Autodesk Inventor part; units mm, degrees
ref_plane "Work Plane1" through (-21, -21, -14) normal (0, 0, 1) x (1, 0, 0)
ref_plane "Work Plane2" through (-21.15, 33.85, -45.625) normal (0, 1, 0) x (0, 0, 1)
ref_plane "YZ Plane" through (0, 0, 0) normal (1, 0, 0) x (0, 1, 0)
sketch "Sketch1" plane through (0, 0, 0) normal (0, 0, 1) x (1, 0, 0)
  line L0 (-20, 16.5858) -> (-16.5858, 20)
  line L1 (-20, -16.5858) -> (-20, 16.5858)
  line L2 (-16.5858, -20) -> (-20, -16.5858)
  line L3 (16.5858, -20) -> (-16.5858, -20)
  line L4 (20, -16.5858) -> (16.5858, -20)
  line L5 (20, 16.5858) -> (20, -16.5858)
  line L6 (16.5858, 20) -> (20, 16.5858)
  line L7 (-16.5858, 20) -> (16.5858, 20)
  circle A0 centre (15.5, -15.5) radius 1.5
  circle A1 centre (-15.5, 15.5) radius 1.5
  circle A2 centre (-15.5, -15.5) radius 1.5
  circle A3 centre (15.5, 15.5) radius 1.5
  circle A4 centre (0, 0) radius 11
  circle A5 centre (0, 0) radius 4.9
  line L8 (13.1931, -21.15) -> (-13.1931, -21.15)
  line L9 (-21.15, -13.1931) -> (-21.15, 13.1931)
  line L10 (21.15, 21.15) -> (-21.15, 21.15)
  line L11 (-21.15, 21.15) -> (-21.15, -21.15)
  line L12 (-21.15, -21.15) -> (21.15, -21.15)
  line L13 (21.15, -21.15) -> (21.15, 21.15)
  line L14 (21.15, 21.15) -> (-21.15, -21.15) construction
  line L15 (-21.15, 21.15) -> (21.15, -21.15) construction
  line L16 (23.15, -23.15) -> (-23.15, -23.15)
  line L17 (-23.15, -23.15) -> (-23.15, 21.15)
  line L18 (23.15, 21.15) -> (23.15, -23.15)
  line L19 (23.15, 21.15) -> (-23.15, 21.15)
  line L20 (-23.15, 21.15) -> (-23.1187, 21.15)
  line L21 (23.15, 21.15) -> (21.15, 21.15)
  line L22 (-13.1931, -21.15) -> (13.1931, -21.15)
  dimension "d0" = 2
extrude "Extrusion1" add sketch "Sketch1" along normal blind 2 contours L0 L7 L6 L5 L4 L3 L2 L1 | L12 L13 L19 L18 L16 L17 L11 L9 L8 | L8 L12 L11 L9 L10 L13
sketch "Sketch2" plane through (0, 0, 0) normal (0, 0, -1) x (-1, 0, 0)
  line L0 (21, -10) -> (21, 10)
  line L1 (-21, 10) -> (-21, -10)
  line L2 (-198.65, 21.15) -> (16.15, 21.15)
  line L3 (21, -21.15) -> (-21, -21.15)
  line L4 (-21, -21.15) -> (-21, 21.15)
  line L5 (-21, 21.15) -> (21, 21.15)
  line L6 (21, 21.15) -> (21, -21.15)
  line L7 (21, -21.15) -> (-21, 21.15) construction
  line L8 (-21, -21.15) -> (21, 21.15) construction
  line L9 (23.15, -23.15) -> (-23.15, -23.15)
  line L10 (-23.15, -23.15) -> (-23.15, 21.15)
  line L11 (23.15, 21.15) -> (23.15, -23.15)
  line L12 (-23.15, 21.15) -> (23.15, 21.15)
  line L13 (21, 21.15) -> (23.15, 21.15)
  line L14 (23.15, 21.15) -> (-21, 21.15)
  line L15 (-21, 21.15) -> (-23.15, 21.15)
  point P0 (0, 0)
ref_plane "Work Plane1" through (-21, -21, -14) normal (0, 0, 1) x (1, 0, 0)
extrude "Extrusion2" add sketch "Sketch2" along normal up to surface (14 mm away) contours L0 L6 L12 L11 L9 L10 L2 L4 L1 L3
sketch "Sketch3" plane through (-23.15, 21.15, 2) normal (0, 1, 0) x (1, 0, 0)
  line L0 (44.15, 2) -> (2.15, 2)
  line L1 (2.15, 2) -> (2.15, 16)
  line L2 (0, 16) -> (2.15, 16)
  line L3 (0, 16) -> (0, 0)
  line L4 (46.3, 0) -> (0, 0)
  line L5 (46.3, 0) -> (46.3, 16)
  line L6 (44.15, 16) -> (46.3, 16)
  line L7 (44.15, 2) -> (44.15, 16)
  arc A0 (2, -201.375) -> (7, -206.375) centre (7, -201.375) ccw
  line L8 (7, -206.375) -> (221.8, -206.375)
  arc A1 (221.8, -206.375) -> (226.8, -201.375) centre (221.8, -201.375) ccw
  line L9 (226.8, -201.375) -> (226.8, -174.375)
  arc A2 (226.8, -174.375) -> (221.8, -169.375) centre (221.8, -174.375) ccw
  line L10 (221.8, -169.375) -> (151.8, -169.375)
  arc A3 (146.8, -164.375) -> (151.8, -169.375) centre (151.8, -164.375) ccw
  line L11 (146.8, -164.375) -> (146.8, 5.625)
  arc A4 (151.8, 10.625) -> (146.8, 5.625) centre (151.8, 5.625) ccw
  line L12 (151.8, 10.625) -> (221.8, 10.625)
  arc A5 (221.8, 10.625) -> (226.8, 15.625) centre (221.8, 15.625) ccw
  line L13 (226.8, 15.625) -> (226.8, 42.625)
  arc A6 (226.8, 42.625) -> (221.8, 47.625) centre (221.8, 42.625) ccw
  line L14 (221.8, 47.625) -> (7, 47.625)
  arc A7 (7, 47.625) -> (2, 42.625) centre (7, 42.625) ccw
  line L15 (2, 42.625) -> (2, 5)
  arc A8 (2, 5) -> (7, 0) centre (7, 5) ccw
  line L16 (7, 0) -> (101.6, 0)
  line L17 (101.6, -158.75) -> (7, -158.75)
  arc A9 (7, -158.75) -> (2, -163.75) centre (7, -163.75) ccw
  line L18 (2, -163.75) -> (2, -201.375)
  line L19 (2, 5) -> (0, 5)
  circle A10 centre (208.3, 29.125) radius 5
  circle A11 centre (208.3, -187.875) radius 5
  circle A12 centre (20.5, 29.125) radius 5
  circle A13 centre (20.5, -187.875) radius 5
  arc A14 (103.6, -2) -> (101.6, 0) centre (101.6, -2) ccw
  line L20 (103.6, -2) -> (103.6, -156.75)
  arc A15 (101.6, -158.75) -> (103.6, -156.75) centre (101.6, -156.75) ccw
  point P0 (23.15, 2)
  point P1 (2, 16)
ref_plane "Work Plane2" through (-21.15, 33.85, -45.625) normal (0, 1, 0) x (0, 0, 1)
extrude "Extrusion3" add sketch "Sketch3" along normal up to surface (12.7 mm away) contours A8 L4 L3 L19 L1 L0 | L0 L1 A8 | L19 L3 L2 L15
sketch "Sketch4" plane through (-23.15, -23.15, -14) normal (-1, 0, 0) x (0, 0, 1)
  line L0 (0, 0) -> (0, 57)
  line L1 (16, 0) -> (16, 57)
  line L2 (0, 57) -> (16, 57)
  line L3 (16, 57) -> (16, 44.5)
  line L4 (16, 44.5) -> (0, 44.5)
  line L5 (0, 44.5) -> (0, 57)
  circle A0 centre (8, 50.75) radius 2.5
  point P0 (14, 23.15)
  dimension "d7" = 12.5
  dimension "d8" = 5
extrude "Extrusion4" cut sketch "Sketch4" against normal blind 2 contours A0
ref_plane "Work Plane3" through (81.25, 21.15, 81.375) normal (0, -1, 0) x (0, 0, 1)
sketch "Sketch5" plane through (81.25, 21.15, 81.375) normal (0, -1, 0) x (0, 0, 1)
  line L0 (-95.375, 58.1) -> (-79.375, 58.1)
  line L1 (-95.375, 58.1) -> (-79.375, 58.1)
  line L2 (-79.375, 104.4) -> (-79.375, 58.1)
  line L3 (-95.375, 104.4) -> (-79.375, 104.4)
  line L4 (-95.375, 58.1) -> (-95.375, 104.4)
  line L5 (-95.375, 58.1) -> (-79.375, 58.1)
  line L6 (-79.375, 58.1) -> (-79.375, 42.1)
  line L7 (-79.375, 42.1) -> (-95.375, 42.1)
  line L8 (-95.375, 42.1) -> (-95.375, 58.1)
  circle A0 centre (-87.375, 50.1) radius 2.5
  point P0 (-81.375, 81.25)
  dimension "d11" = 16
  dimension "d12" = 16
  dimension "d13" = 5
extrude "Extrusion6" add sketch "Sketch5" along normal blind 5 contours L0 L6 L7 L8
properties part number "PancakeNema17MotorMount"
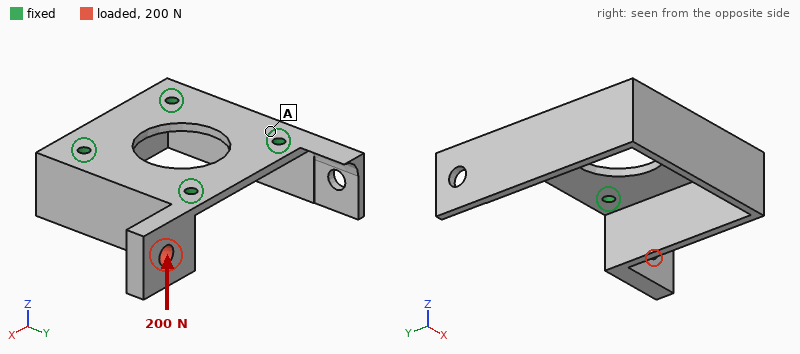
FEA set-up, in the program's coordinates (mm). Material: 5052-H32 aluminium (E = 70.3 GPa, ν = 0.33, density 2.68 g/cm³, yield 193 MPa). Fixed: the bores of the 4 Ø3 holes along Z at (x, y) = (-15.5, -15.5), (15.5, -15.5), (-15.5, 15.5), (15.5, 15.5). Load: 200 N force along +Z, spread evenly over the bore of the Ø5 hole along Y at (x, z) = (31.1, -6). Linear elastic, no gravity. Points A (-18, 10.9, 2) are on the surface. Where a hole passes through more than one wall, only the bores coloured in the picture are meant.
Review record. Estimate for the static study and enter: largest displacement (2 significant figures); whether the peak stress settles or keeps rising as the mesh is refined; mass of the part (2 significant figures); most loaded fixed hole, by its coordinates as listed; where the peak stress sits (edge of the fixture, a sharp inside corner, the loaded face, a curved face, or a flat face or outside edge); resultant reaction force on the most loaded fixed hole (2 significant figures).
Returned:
0.41 mm
keeps rising
23 g
(15.5, 15.5)
edge of the fixture
220 N
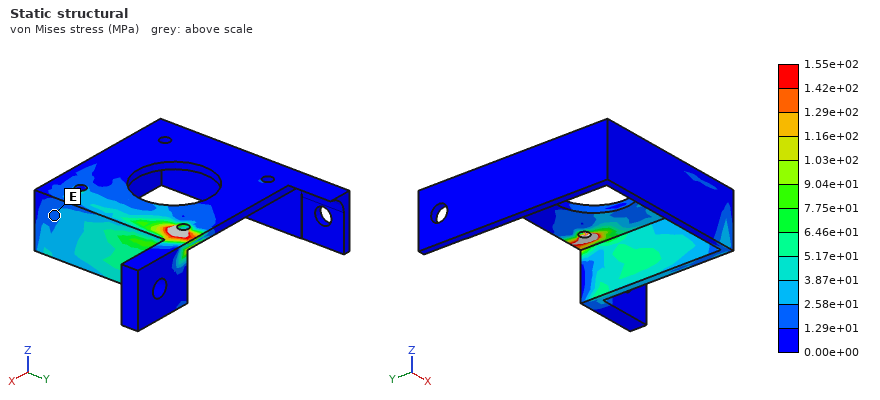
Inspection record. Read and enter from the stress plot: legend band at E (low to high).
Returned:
1.29e+01 to 2.58e+01 MPa
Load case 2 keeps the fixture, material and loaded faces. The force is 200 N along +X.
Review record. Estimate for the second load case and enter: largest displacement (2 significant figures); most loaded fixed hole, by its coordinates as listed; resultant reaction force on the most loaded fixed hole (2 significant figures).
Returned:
0.23 mm
(15.5, 15.5)
200 N
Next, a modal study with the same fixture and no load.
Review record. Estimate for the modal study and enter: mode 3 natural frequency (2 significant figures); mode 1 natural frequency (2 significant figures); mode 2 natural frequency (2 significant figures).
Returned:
5800 Hz
2100 Hz
3900 Hz
